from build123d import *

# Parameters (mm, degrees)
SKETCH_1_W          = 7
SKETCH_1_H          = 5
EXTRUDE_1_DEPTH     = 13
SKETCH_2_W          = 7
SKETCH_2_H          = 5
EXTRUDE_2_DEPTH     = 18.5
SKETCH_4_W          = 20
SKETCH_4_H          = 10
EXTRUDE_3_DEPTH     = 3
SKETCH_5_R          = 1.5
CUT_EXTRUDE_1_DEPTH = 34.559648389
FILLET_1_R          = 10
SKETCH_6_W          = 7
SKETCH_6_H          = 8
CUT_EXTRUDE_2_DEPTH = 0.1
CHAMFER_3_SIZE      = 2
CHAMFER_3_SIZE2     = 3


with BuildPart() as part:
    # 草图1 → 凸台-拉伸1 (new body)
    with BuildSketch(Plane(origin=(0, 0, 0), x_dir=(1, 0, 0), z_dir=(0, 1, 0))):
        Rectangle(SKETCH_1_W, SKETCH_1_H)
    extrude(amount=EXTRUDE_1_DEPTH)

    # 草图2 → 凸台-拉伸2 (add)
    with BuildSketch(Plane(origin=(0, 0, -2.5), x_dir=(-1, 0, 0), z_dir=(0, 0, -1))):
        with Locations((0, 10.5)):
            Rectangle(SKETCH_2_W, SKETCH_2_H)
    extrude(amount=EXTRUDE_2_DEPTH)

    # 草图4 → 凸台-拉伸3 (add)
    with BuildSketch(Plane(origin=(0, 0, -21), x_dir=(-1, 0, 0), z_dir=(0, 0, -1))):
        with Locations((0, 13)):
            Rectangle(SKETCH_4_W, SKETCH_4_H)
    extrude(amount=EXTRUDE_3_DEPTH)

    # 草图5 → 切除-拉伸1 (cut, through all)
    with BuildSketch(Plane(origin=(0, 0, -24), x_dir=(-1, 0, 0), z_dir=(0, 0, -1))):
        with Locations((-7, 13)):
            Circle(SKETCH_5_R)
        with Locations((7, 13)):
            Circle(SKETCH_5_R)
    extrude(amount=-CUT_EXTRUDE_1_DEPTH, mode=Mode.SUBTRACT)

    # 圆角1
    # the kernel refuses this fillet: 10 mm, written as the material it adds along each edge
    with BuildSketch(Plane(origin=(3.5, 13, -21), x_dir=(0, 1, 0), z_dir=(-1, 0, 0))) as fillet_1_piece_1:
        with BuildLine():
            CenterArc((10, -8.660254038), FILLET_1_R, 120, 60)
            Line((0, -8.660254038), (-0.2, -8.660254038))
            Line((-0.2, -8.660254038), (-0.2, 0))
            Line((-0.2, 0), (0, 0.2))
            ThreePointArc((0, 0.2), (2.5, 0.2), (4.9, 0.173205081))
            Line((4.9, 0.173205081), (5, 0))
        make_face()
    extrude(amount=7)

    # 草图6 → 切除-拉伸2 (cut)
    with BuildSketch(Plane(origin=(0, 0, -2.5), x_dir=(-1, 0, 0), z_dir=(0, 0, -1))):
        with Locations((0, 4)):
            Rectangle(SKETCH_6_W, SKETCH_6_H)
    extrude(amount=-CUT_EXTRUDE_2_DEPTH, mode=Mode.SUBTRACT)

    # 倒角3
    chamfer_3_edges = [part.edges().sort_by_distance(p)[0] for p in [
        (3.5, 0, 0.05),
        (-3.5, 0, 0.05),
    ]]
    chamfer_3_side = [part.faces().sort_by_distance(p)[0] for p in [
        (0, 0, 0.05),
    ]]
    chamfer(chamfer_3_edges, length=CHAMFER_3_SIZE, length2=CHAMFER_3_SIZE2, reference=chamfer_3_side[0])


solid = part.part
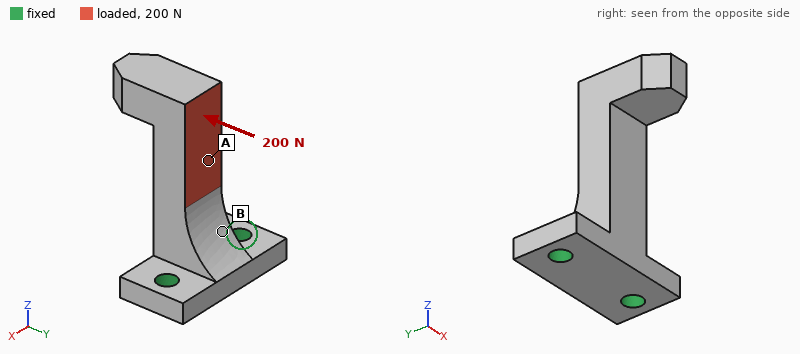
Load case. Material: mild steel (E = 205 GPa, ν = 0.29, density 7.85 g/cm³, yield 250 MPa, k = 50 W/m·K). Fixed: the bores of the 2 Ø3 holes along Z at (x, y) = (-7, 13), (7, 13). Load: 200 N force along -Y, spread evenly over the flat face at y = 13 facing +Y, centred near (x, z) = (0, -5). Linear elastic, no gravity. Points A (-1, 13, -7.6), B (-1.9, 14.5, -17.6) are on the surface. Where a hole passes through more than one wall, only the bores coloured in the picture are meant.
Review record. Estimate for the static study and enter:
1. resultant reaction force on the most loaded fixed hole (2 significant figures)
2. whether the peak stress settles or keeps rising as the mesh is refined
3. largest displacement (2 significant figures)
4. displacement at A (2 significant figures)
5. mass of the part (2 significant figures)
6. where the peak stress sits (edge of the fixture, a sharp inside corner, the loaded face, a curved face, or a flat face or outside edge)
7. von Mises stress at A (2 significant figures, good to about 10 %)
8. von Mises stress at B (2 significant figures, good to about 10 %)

100 N
keeps rising
51 µm
22 µm
13 g
edge of the fixture
24 MPa
62 MPa
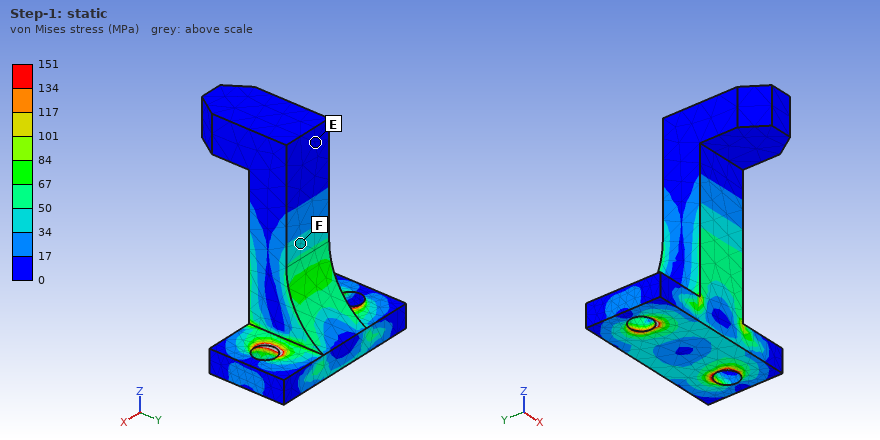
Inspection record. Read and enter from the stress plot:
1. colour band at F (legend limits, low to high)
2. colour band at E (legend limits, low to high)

34 to 50 MPa
0 to 17 MPa
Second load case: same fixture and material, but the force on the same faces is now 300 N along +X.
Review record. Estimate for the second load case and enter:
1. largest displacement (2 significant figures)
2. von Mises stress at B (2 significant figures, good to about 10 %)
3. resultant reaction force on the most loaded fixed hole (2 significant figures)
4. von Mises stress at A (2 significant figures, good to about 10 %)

37 µm
62 MPa
530 N
38 MPa
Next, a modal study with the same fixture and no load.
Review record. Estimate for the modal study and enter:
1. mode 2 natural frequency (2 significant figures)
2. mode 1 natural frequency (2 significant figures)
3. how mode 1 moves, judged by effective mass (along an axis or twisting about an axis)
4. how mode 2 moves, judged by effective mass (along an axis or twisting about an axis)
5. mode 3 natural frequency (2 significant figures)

6200 Hz
4400 Hz
along Y
along X
16 kHz
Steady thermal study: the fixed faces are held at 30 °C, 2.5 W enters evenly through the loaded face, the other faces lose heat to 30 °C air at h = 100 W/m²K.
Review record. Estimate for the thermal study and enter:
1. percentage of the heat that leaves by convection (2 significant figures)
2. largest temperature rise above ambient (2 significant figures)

35 %
18 K
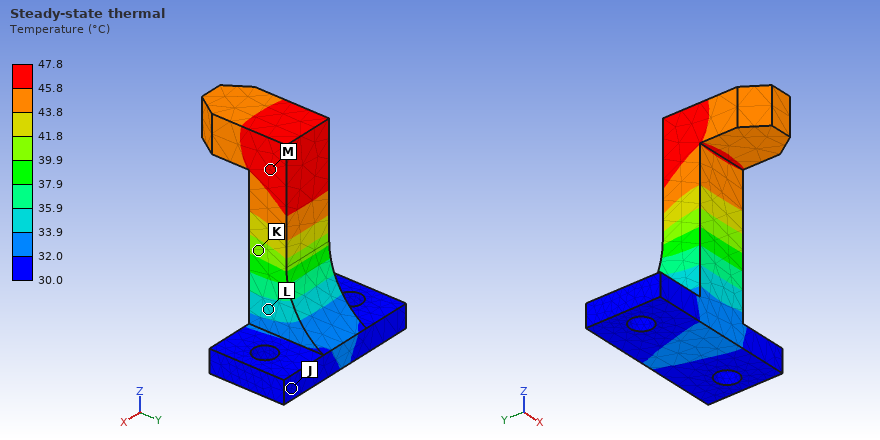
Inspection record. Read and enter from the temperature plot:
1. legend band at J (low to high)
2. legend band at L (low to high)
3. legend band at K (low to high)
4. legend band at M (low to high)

30.0 to 32.0 °C
33.9 to 35.9 °C
39.9 to 41.8 °C
45.8 to 47.8 °C
